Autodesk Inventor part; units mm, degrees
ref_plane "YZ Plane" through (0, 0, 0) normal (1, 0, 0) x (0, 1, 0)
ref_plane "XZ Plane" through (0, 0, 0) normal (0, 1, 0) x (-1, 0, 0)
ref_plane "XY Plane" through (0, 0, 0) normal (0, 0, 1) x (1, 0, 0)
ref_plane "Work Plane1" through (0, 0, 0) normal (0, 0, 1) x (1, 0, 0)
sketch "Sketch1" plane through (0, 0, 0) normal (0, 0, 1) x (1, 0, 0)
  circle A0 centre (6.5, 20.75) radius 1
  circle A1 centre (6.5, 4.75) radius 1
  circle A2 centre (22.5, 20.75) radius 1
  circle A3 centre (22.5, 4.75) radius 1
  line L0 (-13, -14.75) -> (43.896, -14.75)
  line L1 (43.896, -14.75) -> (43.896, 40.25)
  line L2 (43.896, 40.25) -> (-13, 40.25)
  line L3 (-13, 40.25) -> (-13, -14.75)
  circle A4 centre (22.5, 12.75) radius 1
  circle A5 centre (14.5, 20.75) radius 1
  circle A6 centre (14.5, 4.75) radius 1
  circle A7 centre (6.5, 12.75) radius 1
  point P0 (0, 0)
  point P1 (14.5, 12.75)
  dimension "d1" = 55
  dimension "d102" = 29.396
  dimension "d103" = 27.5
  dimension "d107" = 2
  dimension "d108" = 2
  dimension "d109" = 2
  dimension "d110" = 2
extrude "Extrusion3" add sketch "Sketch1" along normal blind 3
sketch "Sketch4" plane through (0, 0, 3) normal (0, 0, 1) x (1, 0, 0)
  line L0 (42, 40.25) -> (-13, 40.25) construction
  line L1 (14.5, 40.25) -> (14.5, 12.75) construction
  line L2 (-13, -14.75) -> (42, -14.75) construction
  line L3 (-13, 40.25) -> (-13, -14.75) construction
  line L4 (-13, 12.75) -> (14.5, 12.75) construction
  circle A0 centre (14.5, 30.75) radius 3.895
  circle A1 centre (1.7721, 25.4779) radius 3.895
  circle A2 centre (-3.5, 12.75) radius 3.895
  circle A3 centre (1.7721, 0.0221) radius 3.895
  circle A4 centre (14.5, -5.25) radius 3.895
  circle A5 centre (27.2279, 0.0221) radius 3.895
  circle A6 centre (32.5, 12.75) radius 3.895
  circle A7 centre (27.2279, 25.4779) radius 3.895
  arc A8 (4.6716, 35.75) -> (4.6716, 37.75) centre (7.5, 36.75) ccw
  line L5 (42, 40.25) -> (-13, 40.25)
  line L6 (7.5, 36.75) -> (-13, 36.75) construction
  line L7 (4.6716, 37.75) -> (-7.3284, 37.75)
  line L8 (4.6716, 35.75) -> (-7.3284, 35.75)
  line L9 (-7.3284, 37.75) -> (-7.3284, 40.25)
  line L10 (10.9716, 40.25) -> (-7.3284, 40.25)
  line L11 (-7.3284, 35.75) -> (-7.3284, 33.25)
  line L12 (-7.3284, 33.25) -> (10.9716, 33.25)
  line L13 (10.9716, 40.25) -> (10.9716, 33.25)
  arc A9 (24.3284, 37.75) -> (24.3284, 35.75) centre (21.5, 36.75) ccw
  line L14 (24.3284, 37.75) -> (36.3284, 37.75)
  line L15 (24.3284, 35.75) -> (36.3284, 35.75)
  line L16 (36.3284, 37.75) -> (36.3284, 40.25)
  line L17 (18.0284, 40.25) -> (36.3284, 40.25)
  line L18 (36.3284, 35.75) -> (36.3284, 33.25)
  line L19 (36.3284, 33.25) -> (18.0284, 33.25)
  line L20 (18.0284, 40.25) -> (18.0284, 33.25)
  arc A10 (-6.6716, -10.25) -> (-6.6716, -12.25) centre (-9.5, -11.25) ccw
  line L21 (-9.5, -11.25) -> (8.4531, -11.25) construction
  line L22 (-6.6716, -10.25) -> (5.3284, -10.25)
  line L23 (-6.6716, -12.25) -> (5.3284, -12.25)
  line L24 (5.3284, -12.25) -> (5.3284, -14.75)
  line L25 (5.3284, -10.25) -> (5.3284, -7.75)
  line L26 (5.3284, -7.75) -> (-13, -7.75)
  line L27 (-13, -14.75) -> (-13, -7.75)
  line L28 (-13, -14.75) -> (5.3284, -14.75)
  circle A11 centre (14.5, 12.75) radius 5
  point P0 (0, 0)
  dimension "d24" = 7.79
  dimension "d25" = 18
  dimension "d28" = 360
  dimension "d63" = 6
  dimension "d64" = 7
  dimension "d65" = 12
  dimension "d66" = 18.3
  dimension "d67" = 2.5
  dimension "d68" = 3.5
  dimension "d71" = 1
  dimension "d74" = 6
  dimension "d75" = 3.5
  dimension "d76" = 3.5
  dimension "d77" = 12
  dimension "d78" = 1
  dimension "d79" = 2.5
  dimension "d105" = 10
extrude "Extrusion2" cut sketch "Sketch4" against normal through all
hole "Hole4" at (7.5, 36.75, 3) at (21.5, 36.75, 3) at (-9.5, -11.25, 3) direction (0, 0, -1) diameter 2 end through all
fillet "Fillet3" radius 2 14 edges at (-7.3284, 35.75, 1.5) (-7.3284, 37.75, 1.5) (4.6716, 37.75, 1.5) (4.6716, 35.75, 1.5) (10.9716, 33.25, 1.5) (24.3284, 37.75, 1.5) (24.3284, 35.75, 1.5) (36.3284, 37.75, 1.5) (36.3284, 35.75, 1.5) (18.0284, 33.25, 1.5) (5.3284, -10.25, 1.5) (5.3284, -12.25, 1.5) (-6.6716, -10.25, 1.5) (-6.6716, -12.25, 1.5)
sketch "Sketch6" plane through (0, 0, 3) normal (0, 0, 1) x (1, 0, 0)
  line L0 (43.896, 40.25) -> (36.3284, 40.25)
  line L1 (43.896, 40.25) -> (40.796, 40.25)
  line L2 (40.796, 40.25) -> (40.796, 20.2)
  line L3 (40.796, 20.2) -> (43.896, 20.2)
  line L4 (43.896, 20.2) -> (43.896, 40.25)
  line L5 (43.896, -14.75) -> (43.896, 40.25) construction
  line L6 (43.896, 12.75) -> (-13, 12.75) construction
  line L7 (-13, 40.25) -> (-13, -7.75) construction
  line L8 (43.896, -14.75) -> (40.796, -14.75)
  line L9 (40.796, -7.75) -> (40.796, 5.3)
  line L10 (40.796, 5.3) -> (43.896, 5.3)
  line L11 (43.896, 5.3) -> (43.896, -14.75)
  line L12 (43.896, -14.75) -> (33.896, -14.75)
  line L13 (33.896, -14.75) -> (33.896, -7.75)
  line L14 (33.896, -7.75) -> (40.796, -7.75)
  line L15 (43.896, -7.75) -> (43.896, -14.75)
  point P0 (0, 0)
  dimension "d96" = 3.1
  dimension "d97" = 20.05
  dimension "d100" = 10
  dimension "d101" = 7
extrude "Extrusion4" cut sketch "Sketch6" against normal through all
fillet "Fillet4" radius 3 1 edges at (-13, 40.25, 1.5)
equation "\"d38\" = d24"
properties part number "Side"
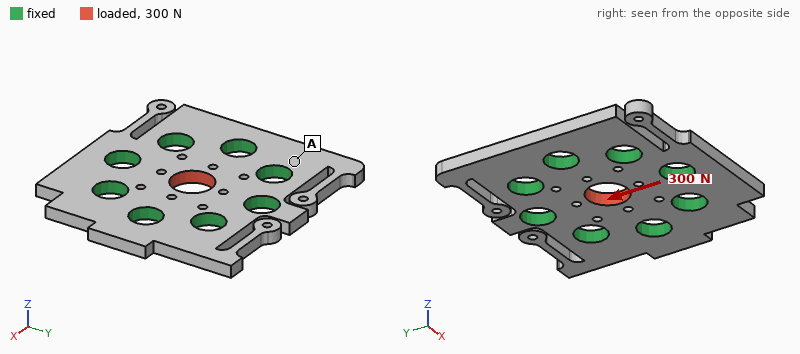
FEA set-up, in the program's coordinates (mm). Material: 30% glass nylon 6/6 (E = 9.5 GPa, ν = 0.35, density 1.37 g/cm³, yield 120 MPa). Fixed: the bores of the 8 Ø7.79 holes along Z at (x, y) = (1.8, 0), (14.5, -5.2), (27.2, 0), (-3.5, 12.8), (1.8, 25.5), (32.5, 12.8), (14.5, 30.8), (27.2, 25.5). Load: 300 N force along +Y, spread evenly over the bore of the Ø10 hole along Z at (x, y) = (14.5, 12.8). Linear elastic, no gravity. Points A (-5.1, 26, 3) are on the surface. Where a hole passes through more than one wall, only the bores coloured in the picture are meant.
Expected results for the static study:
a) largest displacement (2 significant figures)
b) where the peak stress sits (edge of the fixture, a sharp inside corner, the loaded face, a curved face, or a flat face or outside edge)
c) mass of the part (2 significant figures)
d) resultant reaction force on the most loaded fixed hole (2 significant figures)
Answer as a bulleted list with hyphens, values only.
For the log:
- 3.5 µm
- a curved face
- 9.2 g
- 73 N
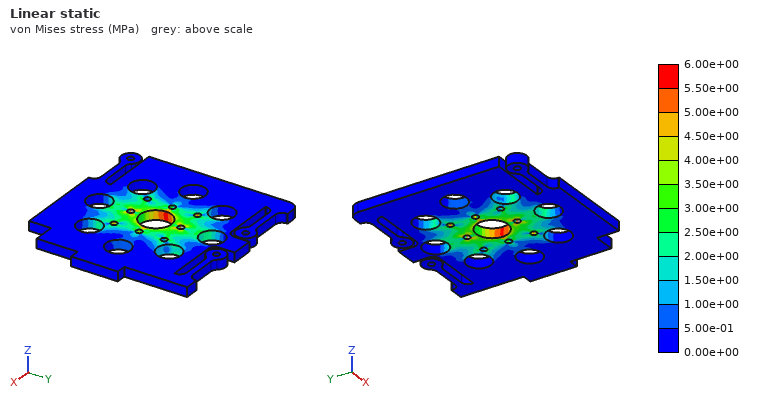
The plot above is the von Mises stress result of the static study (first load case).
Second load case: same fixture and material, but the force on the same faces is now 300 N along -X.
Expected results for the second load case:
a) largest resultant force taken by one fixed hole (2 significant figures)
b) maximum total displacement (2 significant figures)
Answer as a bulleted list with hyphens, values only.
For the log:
- 73 N
- 3.5 µm
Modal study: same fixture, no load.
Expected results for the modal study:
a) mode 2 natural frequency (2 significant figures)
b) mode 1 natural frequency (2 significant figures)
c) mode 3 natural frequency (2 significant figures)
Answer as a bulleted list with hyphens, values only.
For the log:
- 1900 Hz
- 1900 Hz
- 2000 Hz
